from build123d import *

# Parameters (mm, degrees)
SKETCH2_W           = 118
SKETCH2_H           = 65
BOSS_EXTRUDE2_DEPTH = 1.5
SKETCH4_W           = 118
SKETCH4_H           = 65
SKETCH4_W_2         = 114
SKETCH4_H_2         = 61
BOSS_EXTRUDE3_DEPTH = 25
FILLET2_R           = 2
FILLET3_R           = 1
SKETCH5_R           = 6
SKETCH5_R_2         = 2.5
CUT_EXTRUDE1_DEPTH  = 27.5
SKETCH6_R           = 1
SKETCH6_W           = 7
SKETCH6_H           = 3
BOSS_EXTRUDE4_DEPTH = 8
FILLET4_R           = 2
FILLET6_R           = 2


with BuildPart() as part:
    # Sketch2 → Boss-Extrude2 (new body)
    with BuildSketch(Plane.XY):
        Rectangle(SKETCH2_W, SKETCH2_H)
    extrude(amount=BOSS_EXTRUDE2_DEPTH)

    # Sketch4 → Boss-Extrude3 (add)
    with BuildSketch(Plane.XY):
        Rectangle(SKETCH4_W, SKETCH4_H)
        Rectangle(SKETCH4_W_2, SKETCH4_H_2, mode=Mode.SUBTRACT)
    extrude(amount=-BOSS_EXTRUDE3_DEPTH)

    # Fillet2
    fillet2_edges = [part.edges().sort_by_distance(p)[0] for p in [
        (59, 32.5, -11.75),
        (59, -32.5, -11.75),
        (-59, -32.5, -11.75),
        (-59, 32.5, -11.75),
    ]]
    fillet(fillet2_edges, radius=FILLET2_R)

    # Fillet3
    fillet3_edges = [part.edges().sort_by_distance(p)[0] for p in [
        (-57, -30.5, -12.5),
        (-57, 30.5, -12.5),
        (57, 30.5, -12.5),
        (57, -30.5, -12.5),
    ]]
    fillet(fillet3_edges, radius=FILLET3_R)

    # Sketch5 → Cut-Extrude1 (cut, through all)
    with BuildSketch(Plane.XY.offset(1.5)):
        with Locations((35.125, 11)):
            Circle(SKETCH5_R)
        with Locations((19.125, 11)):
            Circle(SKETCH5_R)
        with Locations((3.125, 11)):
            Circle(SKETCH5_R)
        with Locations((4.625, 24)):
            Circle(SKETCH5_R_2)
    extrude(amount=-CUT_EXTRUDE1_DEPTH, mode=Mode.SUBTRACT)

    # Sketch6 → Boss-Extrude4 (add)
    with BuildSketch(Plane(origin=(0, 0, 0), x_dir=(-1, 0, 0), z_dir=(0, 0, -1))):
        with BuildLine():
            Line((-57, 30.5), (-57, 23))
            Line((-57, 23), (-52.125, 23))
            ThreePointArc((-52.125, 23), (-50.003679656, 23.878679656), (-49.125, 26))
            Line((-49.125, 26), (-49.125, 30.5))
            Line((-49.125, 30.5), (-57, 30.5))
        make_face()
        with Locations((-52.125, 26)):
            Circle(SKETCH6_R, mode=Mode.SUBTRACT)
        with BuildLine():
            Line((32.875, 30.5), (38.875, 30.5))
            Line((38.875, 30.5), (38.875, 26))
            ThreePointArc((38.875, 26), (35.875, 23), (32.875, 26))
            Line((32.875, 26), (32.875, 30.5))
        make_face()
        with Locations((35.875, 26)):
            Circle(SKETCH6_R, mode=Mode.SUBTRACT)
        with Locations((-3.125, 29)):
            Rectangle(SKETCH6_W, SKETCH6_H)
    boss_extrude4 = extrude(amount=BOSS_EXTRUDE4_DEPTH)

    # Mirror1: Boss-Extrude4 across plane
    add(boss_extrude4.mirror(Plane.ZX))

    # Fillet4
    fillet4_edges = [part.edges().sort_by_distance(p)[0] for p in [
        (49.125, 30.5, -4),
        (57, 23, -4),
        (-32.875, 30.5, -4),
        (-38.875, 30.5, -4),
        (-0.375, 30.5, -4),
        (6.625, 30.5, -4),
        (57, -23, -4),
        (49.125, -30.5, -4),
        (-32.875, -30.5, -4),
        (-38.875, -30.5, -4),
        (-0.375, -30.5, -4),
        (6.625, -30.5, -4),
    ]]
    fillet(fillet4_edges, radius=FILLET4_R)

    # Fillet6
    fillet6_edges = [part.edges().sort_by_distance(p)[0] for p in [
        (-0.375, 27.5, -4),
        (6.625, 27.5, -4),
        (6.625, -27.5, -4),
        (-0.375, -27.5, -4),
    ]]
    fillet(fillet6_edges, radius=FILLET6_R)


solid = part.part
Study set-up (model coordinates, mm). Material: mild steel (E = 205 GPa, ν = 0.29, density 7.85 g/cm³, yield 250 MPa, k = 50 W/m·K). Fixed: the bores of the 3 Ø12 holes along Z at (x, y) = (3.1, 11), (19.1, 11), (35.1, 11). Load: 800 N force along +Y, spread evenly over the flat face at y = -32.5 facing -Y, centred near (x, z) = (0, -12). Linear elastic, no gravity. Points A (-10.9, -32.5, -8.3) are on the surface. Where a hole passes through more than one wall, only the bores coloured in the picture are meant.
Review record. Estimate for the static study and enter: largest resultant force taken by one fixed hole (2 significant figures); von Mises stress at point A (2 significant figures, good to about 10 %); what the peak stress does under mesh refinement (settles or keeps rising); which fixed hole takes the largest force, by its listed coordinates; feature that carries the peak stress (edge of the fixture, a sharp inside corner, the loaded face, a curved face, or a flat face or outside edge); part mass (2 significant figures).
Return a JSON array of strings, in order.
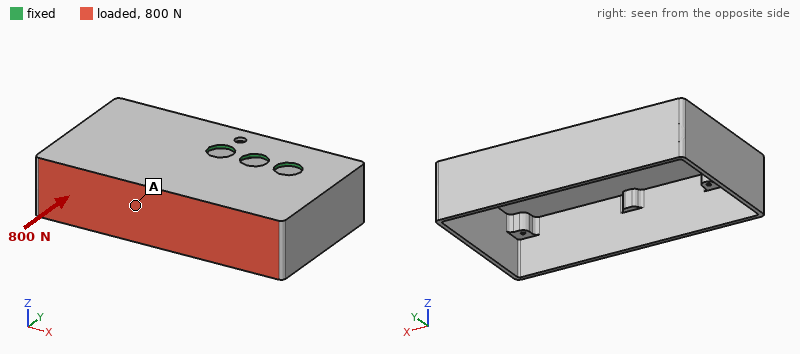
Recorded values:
["730 N", "24 MPa", "keeps rising", "(3.1, 11)", "a sharp inside corner", "240 g"]
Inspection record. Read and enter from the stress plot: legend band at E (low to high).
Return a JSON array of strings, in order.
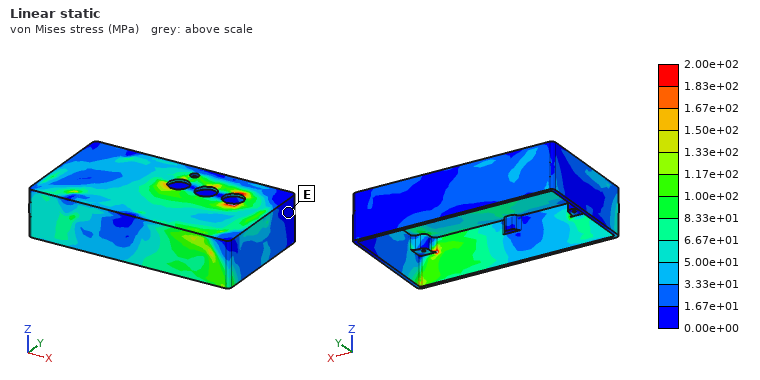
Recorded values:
["0.00e+00 to 1.67e+01 MPa"]
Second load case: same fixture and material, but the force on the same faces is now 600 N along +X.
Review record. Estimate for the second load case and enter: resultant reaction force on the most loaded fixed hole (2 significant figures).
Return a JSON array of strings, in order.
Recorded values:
["600 N"]
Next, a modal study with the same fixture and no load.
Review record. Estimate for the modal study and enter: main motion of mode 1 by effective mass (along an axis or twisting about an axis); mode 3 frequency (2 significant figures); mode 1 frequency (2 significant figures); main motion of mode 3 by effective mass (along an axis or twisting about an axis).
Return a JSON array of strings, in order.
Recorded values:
["along Z", "670 Hz", "320 Hz", "along Z"]
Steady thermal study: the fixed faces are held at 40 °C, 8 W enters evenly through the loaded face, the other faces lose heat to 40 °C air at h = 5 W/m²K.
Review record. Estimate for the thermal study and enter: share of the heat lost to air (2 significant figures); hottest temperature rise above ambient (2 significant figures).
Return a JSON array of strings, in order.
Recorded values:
["29 %", "36 K"]
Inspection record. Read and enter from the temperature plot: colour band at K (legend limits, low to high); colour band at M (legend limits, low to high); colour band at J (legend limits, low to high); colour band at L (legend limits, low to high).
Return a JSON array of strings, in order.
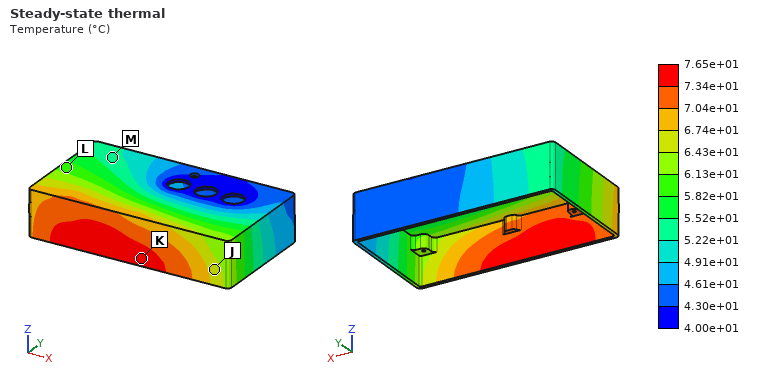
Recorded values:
["7.34e+01 to 7.65e+01 °C", "5.22e+01 to 5.52e+01 °C", "6.43e+01 to 6.74e+01 °C", "5.82e+01 to 6.13e+01 °C"]
